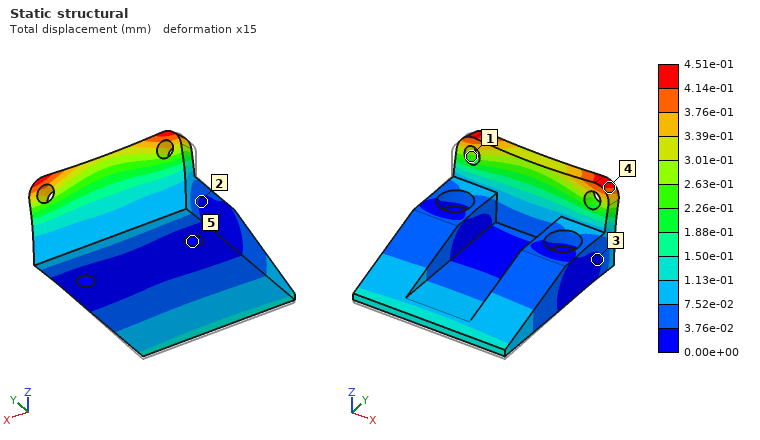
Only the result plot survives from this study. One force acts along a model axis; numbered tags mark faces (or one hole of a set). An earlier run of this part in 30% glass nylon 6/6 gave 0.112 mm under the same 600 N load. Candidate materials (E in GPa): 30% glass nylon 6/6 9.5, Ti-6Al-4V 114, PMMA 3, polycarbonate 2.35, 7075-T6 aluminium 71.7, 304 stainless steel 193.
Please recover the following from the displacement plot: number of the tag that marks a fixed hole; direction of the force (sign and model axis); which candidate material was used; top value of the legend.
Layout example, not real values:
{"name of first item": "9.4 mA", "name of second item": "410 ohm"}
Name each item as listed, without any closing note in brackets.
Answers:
{"number of the tag that marks a fixed hole": "5", "direction of the force": "+Y", "which candidate material was used": "polycarbonate", "top value of the legend": "4.51e-01 mm"}
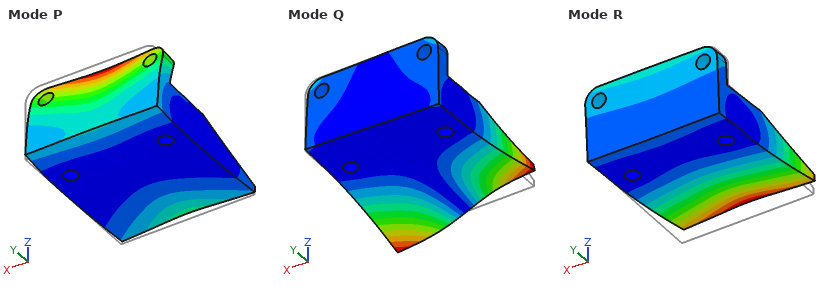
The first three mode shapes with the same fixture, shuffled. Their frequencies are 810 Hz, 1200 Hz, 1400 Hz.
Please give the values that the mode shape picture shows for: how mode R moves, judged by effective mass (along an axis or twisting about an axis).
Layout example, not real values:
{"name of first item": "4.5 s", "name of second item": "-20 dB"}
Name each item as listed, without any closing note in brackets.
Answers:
{"how mode R moves, judged by effective mass": "along Z"}
